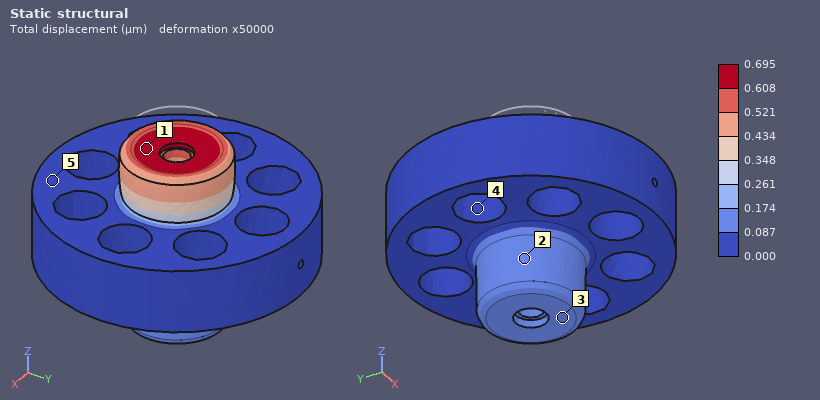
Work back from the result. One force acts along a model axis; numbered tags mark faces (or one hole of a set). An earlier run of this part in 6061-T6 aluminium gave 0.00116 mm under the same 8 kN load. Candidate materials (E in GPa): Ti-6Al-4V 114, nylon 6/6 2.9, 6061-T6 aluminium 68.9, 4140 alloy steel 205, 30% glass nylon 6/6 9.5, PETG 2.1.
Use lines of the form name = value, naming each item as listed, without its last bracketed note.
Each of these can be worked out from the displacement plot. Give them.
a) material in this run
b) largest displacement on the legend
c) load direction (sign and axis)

material in this run = Ti-6Al-4V
largest displacement on the legend = 0.695 µm
load direction = -Z
